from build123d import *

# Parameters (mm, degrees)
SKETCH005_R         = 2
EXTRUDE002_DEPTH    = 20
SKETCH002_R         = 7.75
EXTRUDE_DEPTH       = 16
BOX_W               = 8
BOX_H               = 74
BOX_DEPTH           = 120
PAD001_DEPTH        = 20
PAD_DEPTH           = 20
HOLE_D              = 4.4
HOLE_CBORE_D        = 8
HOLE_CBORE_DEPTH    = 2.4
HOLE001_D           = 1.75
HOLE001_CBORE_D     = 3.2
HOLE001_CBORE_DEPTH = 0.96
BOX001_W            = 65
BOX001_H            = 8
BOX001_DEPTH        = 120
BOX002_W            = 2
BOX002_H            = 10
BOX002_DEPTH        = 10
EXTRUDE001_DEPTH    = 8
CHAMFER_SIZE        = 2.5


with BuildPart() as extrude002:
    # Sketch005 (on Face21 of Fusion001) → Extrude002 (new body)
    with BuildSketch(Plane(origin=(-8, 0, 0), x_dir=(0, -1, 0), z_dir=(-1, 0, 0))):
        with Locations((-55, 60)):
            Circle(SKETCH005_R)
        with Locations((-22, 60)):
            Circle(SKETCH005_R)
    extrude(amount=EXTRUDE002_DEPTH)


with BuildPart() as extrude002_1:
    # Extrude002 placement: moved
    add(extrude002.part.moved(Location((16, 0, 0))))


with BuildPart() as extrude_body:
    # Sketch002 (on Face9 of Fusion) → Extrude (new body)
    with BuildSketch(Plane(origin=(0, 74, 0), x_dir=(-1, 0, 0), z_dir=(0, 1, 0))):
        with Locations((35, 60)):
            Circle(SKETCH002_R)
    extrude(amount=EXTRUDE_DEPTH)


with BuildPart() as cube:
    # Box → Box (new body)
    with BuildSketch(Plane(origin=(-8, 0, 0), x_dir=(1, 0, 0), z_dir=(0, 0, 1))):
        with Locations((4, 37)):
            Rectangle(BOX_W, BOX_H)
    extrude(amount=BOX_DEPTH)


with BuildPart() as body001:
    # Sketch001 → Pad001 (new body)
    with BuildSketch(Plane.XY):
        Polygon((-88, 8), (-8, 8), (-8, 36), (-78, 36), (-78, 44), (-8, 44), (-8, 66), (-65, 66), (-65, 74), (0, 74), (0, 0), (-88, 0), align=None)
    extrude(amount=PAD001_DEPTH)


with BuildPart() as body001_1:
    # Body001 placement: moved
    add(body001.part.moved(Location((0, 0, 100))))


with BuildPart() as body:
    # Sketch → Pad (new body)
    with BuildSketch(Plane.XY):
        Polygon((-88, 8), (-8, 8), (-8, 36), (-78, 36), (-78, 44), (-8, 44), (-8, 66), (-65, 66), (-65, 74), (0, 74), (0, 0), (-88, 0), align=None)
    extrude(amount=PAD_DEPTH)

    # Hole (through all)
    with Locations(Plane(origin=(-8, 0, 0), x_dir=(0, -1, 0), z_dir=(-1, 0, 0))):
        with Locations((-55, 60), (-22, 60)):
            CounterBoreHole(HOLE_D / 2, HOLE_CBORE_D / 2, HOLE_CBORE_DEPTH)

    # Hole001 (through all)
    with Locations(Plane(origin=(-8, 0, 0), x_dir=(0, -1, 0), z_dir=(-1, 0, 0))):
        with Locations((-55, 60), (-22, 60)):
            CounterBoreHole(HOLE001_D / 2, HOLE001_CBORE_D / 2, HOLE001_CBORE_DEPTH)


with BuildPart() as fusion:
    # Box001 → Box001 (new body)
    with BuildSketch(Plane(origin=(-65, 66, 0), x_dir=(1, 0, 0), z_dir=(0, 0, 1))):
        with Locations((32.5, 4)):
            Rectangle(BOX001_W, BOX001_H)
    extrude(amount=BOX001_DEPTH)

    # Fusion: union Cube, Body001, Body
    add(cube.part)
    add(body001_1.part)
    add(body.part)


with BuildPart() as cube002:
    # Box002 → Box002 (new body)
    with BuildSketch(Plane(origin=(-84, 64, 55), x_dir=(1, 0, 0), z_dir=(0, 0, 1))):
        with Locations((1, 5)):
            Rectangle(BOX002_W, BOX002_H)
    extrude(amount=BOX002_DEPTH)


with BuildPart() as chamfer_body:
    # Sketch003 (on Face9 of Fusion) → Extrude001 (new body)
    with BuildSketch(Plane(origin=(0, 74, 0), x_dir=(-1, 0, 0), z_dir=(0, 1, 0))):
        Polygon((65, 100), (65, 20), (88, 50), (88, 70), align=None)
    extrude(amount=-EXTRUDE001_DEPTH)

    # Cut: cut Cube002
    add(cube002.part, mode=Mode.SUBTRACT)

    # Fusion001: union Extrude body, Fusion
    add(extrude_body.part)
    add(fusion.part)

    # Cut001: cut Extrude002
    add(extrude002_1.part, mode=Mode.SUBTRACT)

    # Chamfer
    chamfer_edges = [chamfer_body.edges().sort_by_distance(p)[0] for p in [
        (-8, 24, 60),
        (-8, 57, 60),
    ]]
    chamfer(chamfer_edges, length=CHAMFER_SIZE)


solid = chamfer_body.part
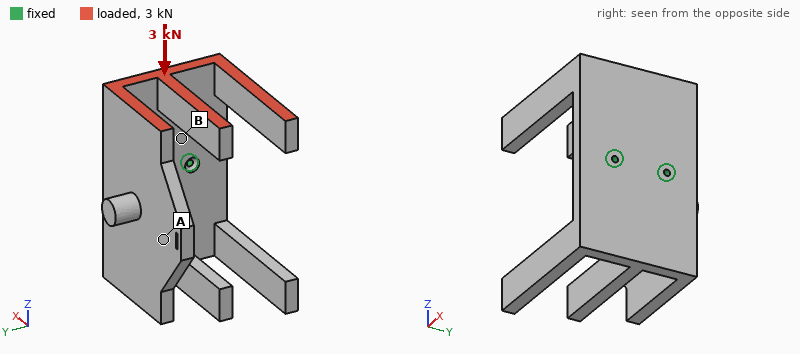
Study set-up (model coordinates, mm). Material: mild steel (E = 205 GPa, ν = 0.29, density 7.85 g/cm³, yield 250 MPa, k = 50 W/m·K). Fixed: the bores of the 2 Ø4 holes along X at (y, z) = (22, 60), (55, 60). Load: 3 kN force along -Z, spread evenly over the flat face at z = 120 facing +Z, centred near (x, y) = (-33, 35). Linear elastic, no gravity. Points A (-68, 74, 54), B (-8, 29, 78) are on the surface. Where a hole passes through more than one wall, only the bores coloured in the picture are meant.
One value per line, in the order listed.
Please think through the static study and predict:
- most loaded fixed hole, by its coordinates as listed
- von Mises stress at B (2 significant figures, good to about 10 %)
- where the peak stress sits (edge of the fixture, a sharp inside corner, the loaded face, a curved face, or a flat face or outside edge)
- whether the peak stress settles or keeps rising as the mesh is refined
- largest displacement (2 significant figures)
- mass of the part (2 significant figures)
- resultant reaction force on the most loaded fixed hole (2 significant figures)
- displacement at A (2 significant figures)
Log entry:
(22, 60)
63 MPa
edge of the fixture
keeps rising
0.65 mm
1.5 kg
1.8 kN
0.17 mm
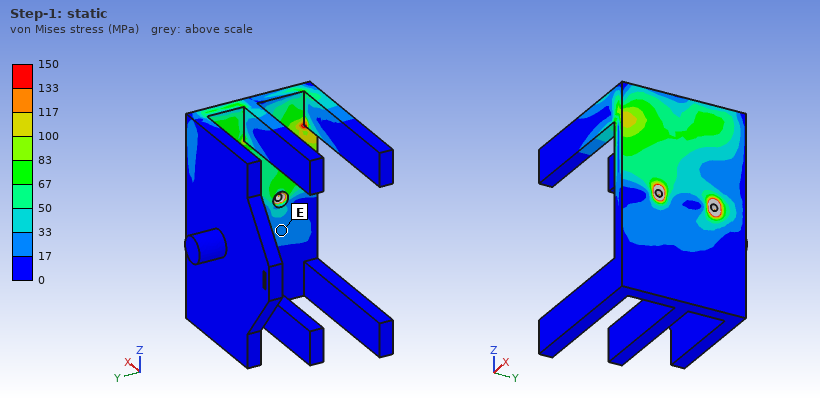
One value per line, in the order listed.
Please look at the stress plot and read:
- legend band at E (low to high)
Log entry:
17 to 33 MPa
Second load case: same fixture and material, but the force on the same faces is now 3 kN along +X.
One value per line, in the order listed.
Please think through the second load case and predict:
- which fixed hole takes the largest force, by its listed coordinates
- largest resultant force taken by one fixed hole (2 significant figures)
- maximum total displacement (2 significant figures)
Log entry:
(22, 60)
1.8 kN
0.85 mm
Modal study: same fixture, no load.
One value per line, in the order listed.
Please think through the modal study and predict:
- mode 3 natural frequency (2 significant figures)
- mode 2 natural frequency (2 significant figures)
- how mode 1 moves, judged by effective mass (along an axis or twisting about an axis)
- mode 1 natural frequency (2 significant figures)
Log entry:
660 Hz
660 Hz
along Z
460 Hz
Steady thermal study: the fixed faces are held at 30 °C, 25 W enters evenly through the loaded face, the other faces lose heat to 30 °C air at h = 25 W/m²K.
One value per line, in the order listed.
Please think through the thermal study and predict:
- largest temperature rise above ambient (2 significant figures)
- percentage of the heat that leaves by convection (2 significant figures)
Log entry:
42 K
57 %
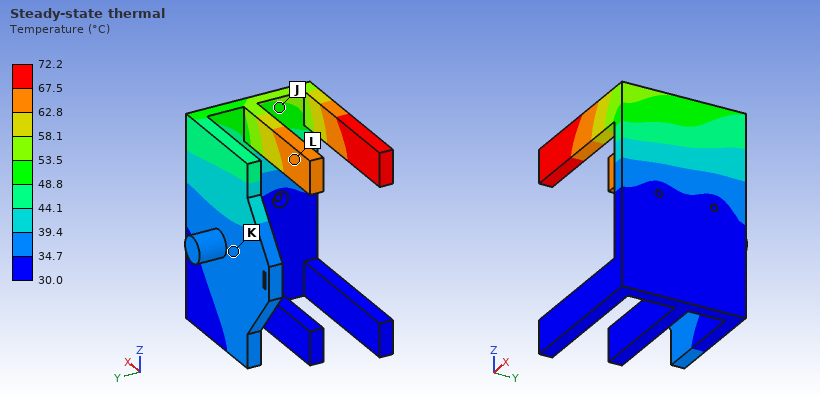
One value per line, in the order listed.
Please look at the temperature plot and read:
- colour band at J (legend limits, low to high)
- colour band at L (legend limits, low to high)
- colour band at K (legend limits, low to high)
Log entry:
48.8 to 53.5 °C
62.8 to 67.5 °C
34.7 to 39.4 °C
